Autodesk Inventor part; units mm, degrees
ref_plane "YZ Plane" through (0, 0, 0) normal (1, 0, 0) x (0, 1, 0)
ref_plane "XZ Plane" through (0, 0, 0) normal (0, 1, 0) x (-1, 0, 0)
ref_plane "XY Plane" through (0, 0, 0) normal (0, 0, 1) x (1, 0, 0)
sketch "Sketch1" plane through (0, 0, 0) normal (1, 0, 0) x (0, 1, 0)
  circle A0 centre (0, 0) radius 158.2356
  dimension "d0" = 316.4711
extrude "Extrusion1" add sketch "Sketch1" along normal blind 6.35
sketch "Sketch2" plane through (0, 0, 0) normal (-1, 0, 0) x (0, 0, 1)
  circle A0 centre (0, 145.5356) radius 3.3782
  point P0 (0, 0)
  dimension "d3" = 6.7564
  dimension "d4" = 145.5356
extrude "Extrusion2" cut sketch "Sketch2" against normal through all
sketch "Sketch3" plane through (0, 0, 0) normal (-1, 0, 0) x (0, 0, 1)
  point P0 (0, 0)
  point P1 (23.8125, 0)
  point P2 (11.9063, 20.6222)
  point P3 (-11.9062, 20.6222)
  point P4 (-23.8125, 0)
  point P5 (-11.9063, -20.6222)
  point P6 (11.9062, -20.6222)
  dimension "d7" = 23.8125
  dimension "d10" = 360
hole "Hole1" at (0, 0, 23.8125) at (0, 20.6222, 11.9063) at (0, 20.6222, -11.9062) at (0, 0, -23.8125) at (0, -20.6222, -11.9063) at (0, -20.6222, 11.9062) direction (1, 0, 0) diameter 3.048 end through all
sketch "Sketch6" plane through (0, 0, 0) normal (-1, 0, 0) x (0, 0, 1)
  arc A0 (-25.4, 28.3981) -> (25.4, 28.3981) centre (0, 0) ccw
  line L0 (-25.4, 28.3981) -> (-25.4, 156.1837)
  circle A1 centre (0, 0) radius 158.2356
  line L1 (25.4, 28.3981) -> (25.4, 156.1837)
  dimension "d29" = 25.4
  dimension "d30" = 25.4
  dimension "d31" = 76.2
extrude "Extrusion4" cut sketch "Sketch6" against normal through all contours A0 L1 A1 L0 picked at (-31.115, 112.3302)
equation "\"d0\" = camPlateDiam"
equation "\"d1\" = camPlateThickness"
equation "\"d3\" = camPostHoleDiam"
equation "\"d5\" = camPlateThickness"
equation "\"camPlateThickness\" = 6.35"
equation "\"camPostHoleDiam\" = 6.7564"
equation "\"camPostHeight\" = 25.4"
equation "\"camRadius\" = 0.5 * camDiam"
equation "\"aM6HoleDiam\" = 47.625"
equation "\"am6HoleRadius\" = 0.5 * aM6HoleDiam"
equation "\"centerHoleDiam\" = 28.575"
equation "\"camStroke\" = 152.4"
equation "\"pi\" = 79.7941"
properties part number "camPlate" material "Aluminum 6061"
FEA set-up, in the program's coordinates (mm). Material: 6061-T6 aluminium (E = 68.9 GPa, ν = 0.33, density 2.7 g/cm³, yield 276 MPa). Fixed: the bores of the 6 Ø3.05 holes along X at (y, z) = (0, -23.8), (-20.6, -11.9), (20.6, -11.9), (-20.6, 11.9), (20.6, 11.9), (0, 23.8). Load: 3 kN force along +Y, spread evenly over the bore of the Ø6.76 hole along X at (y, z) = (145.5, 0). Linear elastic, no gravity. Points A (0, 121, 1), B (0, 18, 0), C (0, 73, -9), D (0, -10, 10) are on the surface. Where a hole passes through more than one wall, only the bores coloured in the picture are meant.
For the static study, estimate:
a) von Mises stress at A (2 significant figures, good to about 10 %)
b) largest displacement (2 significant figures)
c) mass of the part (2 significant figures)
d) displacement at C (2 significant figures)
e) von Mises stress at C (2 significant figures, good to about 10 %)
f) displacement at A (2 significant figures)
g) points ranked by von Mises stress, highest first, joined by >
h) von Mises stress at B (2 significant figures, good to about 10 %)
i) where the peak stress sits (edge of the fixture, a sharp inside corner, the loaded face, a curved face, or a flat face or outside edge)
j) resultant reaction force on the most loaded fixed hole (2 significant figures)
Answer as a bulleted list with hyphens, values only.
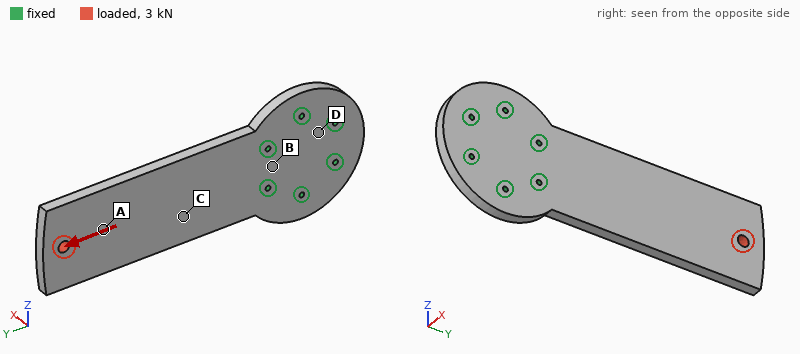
- 13 MPa
- 22 µm
- 180 g
- 7.7 µm
- 9.3 MPa
- 15 µm
- A > C > B > D
- 4.4 MPa
- the loaded face
- 1.1 kN
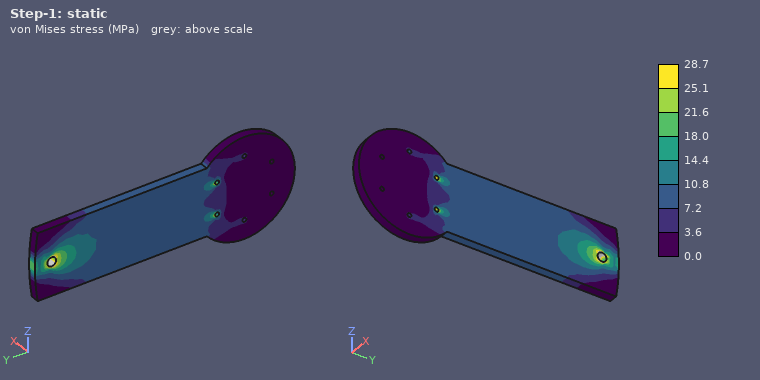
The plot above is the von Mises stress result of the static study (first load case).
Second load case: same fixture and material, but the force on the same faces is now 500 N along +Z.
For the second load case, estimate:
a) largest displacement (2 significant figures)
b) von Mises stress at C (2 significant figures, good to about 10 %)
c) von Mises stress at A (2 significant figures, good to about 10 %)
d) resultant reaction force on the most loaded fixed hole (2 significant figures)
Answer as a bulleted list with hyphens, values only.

- 96 µm
- 6.1 MPa
- 4.0 MPa
- 1.1 kN
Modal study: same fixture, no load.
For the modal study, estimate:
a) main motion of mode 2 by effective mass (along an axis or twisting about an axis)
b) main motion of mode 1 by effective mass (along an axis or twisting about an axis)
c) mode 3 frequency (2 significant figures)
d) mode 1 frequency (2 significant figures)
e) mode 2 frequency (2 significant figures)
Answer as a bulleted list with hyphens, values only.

- twisting about Y
- along X
- 1700 Hz
- 280 Hz
- 1500 Hz
